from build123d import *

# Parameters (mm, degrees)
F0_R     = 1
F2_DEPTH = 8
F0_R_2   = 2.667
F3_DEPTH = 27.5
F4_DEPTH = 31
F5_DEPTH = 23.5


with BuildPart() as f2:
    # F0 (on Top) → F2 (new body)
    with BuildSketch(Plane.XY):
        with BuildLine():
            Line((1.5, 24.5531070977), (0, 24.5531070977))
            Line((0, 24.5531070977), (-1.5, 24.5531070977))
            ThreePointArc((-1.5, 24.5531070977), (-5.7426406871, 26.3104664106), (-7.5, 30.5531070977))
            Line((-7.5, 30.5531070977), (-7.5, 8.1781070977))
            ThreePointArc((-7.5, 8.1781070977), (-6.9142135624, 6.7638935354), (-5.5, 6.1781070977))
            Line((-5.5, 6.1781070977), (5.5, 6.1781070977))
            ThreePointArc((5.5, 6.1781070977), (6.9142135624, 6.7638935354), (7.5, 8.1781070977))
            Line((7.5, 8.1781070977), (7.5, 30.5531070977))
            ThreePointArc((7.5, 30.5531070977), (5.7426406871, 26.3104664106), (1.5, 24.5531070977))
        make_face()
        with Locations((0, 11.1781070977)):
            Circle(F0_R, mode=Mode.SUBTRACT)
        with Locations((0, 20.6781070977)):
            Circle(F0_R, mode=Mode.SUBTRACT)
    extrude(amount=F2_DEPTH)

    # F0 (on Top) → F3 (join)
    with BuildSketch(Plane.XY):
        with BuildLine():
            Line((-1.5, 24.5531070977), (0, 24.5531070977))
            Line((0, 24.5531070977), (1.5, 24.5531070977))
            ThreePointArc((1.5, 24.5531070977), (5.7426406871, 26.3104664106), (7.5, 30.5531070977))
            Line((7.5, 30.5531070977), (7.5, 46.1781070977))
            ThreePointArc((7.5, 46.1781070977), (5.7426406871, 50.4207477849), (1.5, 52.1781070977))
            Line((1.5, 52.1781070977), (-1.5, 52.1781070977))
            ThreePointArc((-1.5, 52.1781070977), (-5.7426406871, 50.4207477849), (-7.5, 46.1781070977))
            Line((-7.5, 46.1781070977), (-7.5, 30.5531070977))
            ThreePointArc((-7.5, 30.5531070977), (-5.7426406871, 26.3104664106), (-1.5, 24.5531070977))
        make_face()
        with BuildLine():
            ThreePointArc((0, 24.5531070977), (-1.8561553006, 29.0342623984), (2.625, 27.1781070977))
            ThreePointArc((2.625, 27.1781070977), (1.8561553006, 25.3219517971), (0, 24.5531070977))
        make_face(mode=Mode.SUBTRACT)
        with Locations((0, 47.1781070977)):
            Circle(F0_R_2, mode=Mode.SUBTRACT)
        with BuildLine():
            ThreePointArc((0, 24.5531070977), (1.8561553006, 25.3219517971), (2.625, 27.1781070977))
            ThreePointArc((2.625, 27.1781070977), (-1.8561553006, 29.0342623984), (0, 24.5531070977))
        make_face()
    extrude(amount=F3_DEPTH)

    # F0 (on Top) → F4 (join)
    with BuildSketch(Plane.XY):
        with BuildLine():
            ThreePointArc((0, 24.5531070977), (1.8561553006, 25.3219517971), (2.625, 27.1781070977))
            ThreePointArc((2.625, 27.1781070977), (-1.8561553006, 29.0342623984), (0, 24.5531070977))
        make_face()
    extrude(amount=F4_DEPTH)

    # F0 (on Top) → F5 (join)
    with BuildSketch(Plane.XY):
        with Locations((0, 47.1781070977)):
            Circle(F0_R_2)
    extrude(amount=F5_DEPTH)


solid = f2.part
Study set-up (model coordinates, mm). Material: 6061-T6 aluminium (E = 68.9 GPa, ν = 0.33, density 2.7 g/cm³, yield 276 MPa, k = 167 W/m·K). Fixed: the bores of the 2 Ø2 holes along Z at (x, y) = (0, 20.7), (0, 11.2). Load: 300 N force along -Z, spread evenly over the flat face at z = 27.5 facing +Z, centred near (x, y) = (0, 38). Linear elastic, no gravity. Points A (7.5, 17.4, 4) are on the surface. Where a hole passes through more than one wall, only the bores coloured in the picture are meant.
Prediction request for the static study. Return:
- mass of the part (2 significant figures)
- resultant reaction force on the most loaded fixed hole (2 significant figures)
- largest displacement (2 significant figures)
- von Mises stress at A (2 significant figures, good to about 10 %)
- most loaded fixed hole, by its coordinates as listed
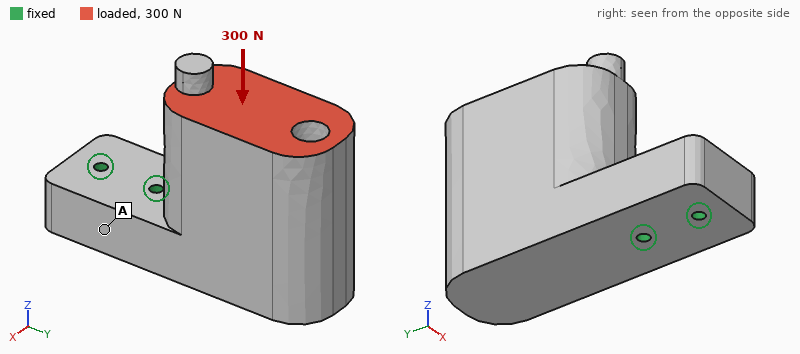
35 g
470 N
39 µm
5.9 MPa
(0, 20.7)
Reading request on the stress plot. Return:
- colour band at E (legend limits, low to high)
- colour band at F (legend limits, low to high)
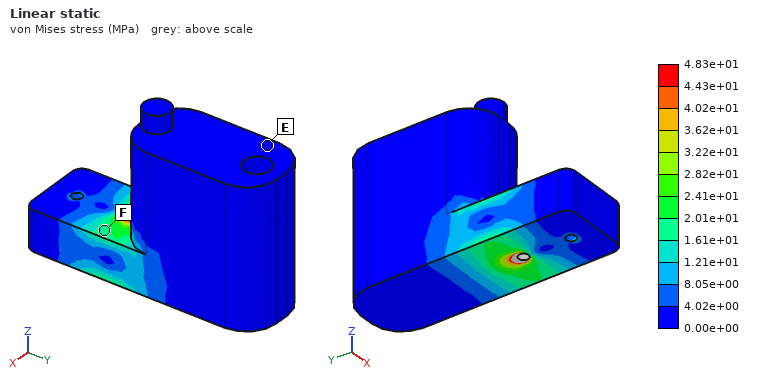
0.00e+00 to 4.02e+00 MPa
1.61e+01 to 2.01e+01 MPa
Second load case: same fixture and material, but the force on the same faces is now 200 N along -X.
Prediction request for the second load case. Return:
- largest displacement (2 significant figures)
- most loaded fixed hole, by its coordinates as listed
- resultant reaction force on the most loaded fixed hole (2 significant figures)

37 µm
(0, 20.7)
500 N
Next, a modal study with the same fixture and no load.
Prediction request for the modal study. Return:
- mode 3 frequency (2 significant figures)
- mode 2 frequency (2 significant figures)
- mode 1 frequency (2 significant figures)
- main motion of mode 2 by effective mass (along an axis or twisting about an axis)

7400 Hz
3700 Hz
3000 Hz
along X
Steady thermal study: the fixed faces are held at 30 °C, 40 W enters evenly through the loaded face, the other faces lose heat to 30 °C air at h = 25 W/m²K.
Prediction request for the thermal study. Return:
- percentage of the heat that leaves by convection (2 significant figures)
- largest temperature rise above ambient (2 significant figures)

4.6 %
37 K
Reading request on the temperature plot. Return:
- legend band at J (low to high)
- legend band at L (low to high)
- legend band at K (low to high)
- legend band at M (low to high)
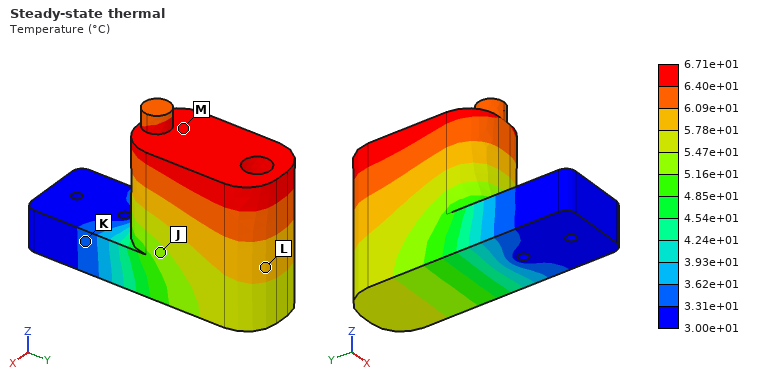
5.16e+01 to 5.47e+01 °C
5.78e+01 to 6.09e+01 °C
3.31e+01 to 3.62e+01 °C
6.40e+01 to 6.71e+01 °C
